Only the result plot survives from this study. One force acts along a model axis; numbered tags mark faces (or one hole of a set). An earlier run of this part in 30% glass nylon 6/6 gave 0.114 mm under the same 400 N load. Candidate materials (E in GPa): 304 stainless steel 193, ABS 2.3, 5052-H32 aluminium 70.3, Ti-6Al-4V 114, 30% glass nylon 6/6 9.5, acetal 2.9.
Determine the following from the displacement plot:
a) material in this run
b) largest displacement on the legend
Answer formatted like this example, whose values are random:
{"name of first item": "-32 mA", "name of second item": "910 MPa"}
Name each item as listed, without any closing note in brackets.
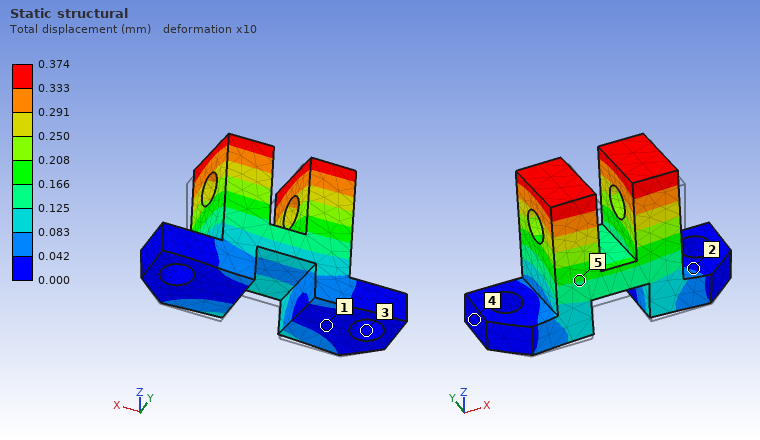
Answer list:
{"material in this run": "acetal", "largest displacement on the legend": "0.374 mm"}
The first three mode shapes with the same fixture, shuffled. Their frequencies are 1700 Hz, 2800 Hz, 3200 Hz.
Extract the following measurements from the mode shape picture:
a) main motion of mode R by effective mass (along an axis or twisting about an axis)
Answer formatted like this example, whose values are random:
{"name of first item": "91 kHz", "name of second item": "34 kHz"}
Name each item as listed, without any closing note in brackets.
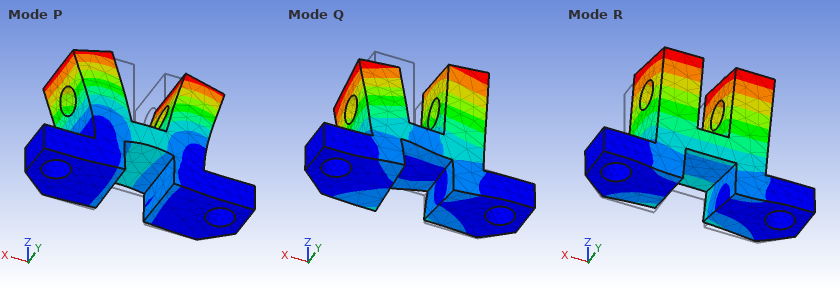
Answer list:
{"main motion of mode R by effective mass": "along Y"}
